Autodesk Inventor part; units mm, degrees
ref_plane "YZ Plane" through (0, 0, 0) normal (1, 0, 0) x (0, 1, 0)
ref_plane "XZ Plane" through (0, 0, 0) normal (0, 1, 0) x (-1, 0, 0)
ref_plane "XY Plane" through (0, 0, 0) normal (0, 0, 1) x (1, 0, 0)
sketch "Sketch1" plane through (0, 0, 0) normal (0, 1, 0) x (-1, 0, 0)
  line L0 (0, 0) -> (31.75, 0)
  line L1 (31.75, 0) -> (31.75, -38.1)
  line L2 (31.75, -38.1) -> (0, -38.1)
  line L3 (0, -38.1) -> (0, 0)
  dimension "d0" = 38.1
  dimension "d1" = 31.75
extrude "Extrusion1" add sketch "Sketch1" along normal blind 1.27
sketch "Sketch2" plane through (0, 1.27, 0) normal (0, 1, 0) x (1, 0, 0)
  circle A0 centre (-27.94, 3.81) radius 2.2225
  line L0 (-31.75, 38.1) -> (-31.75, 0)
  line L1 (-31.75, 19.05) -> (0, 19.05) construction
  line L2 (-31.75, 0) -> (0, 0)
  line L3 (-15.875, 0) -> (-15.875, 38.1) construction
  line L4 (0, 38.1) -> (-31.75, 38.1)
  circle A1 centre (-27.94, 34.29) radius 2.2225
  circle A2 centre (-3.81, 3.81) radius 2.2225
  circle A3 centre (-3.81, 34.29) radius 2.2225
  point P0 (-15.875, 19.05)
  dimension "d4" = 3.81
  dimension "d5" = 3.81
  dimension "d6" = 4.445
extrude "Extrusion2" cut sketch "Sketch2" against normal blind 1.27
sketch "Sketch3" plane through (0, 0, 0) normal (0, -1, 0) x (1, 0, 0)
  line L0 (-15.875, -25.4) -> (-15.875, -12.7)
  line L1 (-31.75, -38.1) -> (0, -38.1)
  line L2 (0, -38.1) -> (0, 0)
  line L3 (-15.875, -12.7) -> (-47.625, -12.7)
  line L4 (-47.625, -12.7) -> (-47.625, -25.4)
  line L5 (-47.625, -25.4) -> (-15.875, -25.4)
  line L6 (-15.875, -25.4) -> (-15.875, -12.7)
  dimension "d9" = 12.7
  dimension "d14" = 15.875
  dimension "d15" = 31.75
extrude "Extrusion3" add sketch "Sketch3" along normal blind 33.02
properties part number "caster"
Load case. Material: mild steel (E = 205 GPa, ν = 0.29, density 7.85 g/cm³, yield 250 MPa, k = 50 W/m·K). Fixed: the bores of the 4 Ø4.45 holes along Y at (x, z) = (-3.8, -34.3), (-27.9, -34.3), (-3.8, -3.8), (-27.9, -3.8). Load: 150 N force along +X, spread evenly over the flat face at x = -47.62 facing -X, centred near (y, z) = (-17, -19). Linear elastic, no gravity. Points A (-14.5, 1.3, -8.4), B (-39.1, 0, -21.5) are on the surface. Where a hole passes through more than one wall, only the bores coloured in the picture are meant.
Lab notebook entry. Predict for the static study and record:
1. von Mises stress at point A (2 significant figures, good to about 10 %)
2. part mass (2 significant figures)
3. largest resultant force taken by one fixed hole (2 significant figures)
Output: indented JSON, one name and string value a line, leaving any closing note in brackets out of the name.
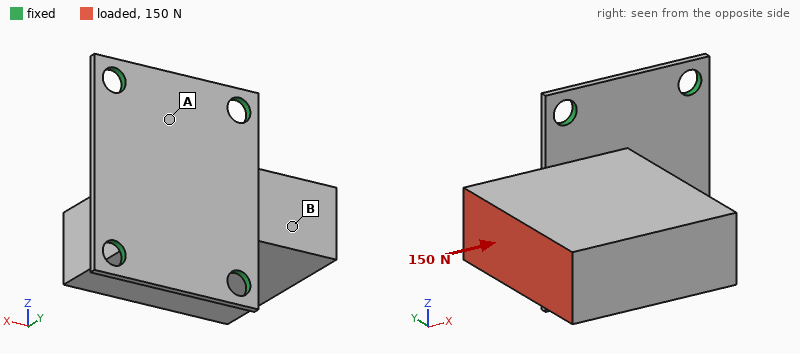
{
  "von Mises stress at point A": "48 MPa",
  "part mass": "120 g",
  "largest resultant force taken by one fixed hole": "81 N"
}
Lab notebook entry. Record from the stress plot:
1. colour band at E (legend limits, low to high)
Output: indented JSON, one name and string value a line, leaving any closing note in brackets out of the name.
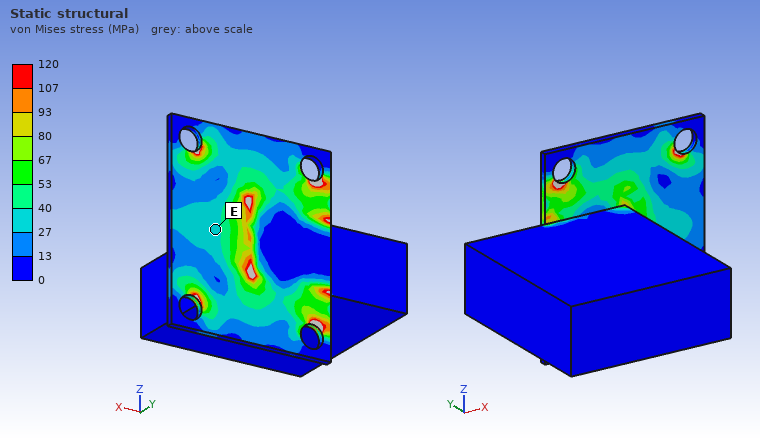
{
  "colour band at E": "27 to 40 MPa"
}
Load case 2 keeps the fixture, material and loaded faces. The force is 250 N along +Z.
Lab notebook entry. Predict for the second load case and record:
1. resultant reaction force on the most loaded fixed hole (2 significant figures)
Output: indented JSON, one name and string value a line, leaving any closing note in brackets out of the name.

{
  "resultant reaction force on the most loaded fixed hole": "240 N"
}
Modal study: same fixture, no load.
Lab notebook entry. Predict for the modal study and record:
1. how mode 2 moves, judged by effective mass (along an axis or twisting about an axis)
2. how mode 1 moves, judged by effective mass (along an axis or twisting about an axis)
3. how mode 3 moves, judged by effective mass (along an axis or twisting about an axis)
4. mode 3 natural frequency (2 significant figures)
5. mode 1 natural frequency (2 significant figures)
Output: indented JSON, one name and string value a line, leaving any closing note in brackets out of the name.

{
  "how mode 2 moves, judged by effective mass": "along Z",
  "how mode 1 moves, judged by effective mass": "along X",
  "how mode 3 moves, judged by effective mass": "along Y",
  "mode 3 natural frequency": "2400 Hz",
  "mode 1 natural frequency": "700 Hz"
}
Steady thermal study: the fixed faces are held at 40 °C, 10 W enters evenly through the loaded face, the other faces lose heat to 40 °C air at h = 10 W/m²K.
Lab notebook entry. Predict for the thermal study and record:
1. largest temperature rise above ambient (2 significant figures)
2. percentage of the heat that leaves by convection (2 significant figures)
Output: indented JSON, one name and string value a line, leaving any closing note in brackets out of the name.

{
  "largest temperature rise above ambient": "50 K",
  "percentage of the heat that leaves by convection": "16 %"
}
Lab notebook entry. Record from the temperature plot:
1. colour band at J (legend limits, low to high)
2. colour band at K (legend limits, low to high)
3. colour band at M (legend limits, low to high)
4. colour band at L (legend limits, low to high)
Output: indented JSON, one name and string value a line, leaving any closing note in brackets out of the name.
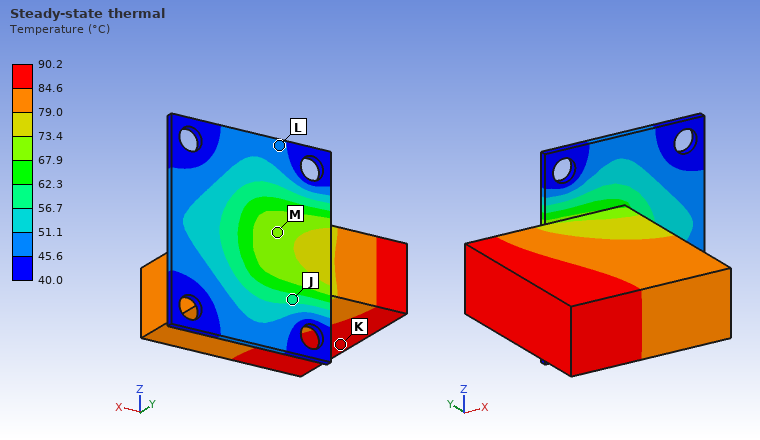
{
  "colour band at J": "56.7 to 62.3 °C",
  "colour band at K": "84.6 to 90.2 °C",
  "colour band at M": "67.9 to 73.4 °C",
  "colour band at L": "45.6 to 51.1 °C"
}
